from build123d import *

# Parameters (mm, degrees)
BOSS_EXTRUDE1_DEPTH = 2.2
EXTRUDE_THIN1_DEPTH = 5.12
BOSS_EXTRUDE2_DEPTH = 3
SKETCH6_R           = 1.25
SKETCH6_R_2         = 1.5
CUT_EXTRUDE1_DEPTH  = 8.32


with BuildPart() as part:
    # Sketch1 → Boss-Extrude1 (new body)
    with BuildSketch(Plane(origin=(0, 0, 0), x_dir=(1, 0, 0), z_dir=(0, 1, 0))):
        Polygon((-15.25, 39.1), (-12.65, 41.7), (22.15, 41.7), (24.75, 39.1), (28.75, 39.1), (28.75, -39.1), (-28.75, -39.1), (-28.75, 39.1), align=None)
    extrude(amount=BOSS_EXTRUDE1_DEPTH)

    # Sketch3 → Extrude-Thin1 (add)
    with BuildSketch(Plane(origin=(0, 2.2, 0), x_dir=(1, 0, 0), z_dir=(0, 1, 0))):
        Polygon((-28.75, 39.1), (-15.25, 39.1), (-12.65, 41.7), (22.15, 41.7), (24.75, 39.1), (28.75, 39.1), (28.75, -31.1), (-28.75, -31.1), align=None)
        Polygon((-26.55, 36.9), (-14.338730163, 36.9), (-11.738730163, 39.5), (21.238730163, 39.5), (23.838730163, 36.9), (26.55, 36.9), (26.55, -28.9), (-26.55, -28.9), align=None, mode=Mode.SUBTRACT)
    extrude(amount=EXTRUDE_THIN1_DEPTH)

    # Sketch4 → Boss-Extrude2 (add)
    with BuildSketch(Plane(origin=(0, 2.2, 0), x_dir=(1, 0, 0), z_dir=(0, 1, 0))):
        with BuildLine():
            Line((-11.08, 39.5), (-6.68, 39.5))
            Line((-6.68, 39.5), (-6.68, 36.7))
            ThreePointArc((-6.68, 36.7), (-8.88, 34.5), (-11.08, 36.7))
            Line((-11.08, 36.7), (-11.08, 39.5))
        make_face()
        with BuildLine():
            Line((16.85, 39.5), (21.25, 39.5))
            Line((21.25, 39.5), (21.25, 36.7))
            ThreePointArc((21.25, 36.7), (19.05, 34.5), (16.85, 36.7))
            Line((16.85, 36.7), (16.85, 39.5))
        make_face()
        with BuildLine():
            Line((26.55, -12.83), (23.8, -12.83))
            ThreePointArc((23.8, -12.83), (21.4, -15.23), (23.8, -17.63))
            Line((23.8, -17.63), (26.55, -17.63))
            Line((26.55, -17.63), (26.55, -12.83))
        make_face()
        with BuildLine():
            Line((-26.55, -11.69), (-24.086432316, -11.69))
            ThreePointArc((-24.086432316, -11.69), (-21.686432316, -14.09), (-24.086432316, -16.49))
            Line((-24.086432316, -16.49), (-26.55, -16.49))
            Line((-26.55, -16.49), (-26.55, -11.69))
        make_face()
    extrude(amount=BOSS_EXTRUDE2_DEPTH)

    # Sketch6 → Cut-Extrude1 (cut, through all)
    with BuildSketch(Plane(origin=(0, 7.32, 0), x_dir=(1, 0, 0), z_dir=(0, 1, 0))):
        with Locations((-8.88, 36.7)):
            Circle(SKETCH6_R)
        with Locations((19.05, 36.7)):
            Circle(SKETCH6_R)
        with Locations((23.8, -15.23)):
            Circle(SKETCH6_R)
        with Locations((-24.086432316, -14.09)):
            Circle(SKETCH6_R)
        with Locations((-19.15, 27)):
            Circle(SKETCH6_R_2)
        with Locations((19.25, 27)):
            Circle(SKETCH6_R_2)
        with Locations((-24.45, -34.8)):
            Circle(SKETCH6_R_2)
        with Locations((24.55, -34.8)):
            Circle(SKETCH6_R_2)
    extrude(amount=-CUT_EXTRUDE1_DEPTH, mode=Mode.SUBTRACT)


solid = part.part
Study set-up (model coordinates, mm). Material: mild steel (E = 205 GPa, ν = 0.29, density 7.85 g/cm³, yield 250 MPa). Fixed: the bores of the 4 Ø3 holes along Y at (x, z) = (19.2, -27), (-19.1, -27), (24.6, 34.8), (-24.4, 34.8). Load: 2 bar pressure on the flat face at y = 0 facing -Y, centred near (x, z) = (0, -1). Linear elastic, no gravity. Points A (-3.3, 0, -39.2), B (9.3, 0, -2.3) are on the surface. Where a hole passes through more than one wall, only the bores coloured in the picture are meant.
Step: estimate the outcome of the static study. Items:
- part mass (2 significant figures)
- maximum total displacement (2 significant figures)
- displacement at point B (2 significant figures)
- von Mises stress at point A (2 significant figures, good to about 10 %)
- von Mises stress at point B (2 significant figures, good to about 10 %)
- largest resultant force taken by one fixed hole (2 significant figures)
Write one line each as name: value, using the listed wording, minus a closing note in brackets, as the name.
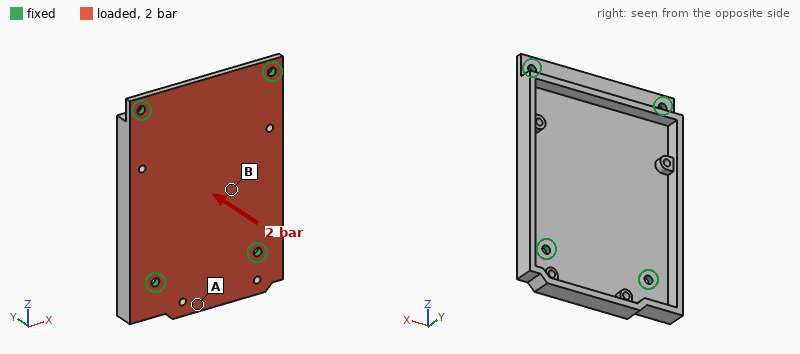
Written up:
part mass: 100 g
maximum total displacement: 37 µm
displacement at point B: 32 µm
von Mises stress at point A: 8.6 MPa
von Mises stress at point B: 25 MPa
largest resultant force taken by one fixed hole: 290 N
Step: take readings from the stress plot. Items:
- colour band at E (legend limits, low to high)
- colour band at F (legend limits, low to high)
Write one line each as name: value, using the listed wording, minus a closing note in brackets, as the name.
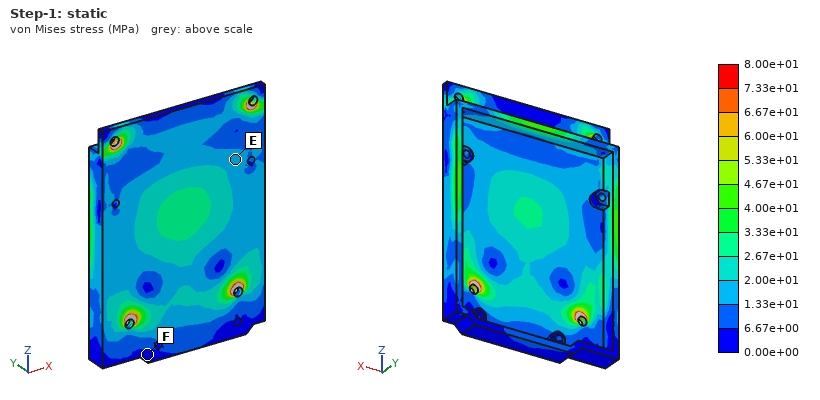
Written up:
colour band at E: 1.33e+01 to 2.00e+01 MPa
colour band at F: 0.00e+00 to 6.67e+00 MPa
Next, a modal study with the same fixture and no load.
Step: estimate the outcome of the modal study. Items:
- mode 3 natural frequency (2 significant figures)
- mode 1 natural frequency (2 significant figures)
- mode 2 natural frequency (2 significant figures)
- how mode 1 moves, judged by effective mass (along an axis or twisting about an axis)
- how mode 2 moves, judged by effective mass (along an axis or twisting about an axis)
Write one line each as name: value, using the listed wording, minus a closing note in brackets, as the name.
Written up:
mode 3 natural frequency: 5700 Hz
mode 1 natural frequency: 3300 Hz
mode 2 natural frequency: 5200 Hz
how mode 1 moves, judged by effective mass: along Y
how mode 2 moves, judged by effective mass: twisting about Z
